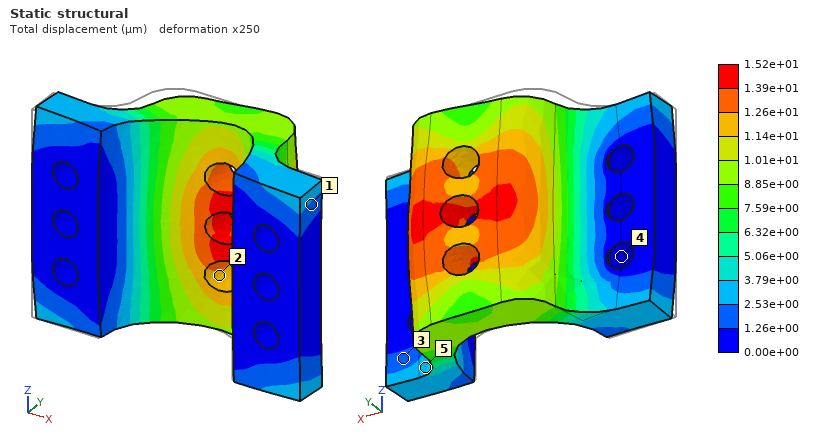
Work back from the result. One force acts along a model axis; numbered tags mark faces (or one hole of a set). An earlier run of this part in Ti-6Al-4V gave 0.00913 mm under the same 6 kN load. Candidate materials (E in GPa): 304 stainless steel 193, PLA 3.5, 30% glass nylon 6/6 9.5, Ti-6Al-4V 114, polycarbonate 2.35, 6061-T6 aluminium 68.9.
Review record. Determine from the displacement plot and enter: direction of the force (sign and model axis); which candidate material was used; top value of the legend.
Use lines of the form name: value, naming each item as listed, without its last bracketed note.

direction of the force: +X
which candidate material was used: 6061-T6 aluminium
top value of the legend: 1.52e+01 µm
